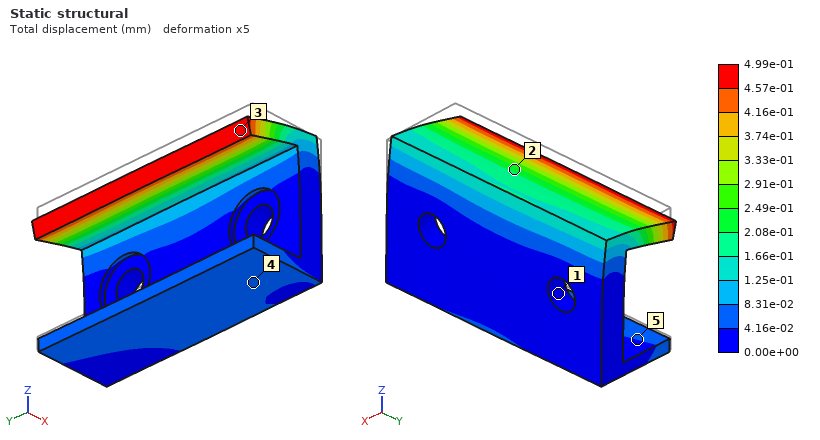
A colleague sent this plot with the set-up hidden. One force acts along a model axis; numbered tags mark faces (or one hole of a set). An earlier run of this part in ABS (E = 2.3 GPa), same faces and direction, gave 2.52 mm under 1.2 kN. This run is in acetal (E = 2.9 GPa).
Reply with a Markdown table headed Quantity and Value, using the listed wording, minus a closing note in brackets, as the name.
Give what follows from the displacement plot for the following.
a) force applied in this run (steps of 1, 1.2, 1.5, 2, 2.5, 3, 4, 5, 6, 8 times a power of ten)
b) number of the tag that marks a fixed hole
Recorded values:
| Quantity | Value |
|---|---|
| force applied in this run | 300 N |
| number of the tag that marks a fixed hole | 1 |
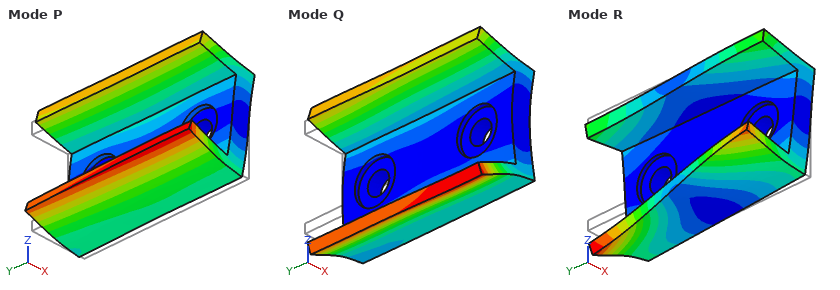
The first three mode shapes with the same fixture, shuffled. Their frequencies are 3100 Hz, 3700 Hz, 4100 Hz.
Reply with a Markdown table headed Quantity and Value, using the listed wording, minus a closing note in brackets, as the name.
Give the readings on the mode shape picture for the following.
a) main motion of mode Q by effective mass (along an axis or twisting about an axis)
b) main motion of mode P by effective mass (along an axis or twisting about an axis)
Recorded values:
| Quantity | Value |
|---|---|
| main motion of mode Q by effective mass | along X |
| main motion of mode P by effective mass | along Z |
